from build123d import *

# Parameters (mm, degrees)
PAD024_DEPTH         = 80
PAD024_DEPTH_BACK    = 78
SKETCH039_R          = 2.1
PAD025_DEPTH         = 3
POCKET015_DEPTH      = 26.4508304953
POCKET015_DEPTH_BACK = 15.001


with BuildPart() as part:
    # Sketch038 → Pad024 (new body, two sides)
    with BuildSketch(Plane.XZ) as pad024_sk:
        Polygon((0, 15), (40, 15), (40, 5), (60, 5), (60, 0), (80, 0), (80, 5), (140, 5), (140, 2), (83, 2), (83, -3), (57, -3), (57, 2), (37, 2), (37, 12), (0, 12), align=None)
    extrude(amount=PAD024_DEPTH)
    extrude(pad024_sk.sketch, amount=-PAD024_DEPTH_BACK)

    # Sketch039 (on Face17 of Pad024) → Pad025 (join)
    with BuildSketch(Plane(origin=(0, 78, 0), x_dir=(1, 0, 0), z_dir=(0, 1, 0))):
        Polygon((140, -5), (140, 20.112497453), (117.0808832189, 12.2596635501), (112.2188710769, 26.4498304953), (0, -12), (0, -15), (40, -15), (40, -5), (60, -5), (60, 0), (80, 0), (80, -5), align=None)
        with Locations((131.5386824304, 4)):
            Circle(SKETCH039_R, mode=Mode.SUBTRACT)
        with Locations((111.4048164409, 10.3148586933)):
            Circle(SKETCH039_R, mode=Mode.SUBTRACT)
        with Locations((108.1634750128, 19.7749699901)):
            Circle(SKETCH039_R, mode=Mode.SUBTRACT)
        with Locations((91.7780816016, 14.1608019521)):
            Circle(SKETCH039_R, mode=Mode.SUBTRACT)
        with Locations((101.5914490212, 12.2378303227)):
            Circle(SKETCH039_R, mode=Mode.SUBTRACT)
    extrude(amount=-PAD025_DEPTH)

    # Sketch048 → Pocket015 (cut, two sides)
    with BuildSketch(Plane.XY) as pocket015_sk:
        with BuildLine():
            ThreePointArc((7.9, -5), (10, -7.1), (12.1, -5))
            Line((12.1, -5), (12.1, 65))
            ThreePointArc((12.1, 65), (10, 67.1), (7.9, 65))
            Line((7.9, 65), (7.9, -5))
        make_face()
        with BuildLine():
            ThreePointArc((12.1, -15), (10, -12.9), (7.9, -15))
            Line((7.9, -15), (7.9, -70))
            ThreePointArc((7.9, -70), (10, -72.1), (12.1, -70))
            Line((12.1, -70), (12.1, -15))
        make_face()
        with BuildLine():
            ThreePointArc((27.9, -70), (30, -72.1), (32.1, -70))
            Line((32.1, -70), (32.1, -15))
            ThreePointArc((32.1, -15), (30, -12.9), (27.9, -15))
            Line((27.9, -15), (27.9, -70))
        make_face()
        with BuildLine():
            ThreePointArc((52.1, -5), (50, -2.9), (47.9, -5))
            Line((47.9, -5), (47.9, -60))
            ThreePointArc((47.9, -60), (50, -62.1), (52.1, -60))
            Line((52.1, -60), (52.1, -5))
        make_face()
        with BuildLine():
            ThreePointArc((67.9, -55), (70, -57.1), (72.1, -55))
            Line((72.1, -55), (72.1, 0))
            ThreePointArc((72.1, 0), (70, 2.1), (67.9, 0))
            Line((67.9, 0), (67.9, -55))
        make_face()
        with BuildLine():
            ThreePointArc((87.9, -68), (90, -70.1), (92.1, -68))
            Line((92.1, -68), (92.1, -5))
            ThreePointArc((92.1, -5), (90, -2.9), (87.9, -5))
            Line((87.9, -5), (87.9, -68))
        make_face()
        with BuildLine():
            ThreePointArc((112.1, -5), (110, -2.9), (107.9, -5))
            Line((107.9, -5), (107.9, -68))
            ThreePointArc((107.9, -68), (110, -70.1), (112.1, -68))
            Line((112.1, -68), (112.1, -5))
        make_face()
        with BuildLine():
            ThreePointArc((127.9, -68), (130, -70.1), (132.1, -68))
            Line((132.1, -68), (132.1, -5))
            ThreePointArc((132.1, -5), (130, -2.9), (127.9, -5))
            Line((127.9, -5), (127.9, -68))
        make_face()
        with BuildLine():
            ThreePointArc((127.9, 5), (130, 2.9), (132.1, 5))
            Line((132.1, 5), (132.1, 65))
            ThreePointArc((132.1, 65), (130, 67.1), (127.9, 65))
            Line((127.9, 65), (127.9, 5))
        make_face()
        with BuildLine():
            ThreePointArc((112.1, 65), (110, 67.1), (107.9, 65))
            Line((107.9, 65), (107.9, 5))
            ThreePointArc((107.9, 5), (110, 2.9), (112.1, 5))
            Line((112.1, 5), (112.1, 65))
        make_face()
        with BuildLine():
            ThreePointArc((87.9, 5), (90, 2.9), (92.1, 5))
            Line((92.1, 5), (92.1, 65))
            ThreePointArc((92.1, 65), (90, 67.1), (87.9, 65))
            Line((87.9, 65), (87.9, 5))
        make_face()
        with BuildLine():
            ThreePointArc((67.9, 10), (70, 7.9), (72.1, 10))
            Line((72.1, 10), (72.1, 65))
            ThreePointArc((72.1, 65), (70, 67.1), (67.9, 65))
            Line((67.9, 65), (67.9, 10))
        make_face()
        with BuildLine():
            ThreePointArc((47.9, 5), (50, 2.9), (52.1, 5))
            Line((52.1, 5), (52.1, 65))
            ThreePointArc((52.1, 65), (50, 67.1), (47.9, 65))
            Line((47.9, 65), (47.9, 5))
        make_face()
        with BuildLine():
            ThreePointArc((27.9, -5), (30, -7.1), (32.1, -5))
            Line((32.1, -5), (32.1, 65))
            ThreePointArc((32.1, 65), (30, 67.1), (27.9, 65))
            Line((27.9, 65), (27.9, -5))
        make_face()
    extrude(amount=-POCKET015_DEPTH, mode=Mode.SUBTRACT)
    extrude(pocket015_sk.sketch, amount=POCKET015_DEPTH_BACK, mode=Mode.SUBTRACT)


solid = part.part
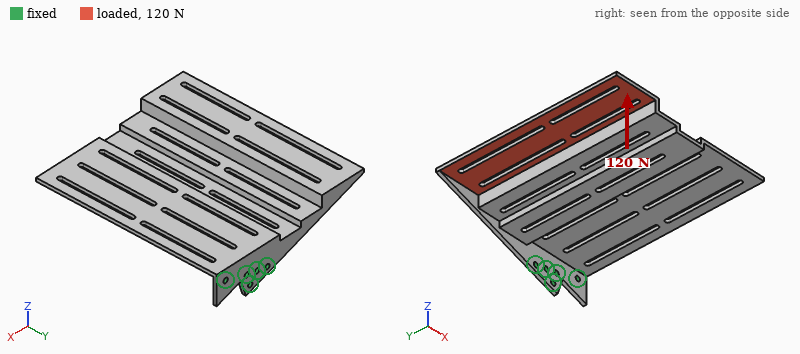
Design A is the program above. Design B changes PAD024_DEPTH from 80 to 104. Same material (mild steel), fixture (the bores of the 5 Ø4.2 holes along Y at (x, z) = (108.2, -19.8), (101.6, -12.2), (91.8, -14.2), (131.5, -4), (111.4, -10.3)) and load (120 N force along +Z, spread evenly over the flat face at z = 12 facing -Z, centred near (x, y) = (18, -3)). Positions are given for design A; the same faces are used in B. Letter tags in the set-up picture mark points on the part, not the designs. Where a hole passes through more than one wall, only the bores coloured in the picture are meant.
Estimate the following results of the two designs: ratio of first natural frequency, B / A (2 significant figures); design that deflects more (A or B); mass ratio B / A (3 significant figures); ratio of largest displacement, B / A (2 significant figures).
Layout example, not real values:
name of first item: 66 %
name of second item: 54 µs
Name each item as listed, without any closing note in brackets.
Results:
ratio of first natural frequency, B / A: 0.79
design that deflects more: B
mass ratio B / A: 1.17
ratio of largest displacement, B / A: 1.3
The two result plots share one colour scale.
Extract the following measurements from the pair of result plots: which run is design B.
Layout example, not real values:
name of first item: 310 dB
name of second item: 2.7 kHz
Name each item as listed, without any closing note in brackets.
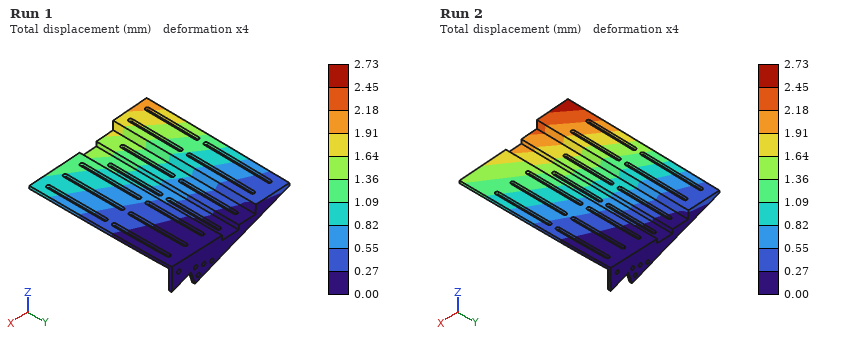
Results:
which run is design B: Run 2
